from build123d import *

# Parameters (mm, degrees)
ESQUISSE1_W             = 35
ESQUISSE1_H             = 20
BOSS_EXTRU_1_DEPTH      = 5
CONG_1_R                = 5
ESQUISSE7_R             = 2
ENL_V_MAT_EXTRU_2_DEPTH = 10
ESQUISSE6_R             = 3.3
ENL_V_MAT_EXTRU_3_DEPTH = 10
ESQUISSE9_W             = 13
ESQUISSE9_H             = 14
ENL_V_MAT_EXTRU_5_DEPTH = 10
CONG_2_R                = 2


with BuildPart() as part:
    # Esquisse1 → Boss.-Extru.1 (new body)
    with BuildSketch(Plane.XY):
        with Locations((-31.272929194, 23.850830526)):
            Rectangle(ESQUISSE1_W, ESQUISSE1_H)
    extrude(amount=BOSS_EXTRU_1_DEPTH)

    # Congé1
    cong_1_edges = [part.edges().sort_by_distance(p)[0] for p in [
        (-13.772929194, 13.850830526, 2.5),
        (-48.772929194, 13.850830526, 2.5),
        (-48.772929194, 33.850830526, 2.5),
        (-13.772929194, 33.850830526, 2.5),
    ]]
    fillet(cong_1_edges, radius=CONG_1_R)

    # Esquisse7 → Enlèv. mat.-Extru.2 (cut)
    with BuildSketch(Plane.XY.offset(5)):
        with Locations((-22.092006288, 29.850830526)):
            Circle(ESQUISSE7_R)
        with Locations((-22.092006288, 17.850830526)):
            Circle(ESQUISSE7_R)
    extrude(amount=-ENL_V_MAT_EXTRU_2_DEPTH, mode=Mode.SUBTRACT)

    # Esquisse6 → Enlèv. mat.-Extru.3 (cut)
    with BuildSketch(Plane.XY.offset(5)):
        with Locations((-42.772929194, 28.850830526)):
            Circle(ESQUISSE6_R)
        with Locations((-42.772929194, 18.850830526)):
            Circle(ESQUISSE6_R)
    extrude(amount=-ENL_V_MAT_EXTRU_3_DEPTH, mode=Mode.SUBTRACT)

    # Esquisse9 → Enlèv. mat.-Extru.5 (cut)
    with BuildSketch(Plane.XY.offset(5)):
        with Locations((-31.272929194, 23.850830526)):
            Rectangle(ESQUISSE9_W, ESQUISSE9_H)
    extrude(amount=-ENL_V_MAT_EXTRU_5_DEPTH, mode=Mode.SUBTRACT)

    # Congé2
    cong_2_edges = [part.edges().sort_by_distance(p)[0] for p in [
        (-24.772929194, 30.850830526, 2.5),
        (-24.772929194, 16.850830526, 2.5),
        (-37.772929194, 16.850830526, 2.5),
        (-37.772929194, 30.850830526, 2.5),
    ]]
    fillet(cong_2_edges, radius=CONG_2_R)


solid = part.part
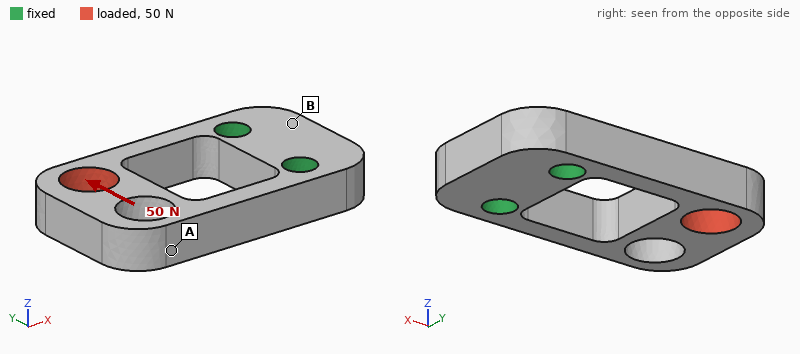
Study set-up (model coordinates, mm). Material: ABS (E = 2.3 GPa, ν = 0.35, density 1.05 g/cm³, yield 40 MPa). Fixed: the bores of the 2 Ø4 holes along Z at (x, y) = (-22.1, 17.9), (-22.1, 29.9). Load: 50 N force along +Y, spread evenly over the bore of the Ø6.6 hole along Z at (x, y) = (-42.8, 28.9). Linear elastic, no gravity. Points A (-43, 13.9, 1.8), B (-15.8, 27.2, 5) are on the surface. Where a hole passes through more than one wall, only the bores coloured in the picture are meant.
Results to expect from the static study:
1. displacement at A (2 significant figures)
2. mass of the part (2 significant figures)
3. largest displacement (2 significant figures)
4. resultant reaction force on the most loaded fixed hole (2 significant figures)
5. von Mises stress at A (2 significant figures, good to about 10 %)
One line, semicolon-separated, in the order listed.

0.38 mm; 2.1 g; 0.40 mm; 47 N; 5.1 MPa
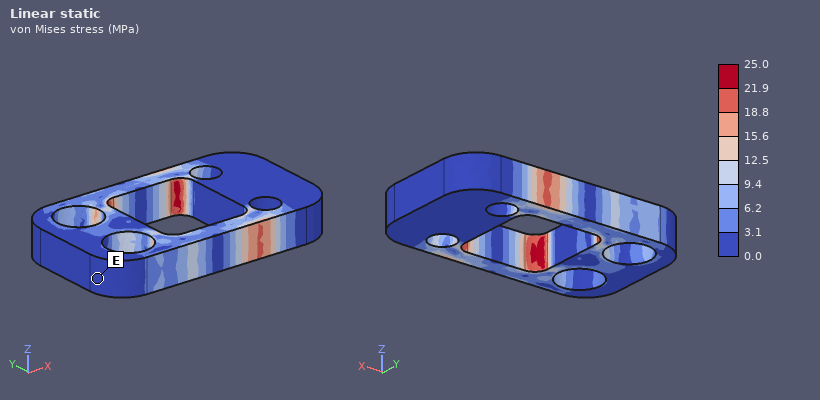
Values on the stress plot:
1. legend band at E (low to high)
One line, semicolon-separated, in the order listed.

0.0 to 3.1 MPa
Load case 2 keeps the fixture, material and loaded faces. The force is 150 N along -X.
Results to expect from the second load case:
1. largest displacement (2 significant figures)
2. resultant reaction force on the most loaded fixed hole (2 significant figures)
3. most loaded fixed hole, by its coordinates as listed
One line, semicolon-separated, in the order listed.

0.12 mm; 120 N; (-22.1, 29.9)
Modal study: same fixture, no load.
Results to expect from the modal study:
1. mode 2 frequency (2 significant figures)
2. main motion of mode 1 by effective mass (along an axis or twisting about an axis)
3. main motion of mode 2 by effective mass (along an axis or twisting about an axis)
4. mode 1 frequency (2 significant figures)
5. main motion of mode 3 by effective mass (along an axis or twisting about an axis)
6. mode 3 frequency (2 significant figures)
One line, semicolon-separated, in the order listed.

2000 Hz; along Z; along Y; 1300 Hz; twisting about X; 3200 Hz
